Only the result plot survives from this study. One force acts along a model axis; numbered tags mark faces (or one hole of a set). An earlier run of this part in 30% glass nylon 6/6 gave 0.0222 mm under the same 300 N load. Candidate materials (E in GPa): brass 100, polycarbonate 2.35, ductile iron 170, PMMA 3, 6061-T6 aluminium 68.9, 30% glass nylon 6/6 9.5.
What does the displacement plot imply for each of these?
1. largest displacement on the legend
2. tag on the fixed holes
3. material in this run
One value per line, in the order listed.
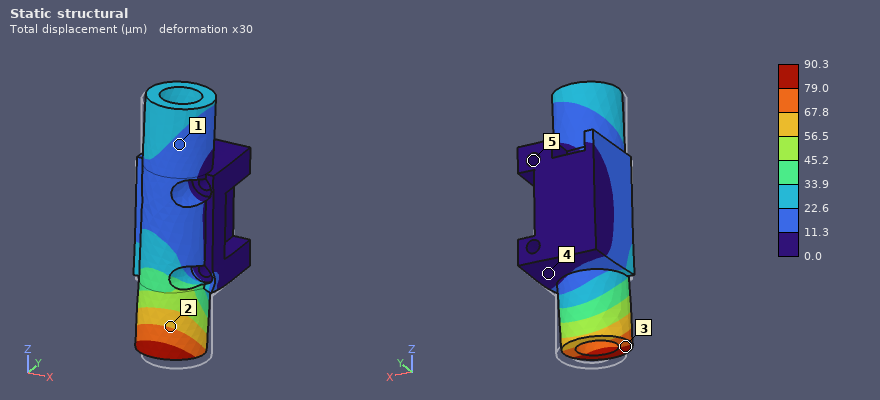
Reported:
90.3 µm
5
polycarbonate
